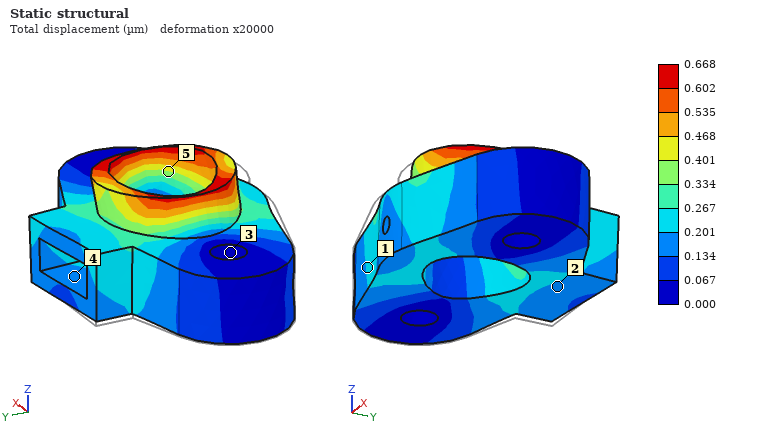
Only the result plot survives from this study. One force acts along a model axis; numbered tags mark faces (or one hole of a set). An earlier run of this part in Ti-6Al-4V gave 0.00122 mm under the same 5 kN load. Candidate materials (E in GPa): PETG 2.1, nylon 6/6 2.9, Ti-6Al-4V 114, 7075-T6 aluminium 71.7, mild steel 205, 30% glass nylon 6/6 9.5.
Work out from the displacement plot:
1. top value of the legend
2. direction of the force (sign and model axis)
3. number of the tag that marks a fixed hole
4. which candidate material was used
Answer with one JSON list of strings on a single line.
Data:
["0.668 µm", "+X", "3", "mild steel"]
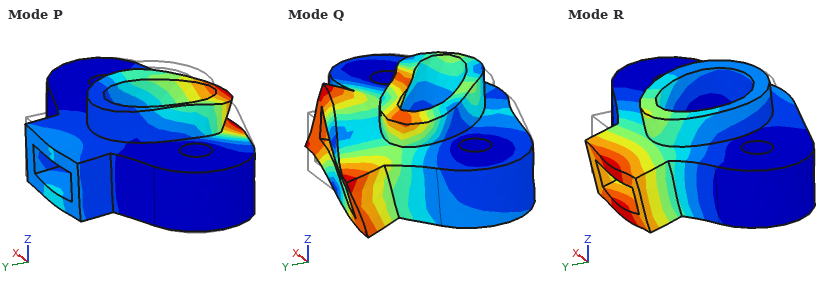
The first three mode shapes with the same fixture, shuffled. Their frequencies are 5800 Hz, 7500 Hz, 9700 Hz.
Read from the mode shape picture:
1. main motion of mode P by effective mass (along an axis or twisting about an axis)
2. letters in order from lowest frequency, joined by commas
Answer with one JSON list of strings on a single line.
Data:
["along Z", "R, P, Q"]
